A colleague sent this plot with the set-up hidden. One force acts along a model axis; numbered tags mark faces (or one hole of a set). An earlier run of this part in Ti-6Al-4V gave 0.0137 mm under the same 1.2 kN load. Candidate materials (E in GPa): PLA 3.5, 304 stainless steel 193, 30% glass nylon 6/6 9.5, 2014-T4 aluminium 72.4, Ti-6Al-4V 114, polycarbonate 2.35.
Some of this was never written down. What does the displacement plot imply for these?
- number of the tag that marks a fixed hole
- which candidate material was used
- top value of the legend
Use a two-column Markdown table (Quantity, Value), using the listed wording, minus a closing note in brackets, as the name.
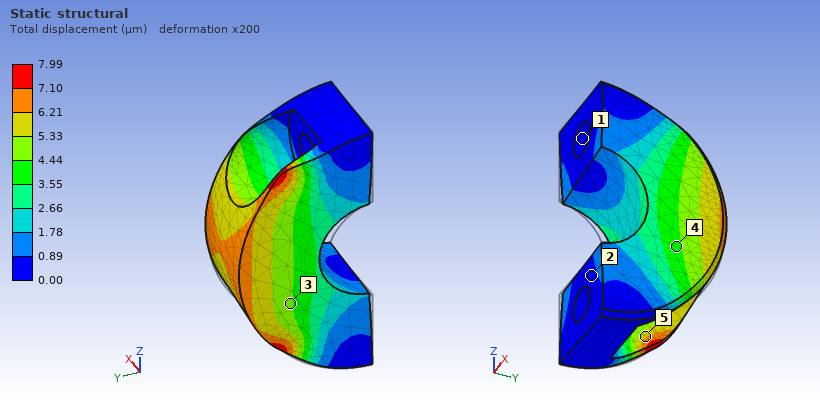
| Quantity | Value |
|---|---|
| number of the tag that marks a fixed hole | 1 |
| which candidate material was used | 304 stainless steel |
| top value of the legend | 7.99 µm |
